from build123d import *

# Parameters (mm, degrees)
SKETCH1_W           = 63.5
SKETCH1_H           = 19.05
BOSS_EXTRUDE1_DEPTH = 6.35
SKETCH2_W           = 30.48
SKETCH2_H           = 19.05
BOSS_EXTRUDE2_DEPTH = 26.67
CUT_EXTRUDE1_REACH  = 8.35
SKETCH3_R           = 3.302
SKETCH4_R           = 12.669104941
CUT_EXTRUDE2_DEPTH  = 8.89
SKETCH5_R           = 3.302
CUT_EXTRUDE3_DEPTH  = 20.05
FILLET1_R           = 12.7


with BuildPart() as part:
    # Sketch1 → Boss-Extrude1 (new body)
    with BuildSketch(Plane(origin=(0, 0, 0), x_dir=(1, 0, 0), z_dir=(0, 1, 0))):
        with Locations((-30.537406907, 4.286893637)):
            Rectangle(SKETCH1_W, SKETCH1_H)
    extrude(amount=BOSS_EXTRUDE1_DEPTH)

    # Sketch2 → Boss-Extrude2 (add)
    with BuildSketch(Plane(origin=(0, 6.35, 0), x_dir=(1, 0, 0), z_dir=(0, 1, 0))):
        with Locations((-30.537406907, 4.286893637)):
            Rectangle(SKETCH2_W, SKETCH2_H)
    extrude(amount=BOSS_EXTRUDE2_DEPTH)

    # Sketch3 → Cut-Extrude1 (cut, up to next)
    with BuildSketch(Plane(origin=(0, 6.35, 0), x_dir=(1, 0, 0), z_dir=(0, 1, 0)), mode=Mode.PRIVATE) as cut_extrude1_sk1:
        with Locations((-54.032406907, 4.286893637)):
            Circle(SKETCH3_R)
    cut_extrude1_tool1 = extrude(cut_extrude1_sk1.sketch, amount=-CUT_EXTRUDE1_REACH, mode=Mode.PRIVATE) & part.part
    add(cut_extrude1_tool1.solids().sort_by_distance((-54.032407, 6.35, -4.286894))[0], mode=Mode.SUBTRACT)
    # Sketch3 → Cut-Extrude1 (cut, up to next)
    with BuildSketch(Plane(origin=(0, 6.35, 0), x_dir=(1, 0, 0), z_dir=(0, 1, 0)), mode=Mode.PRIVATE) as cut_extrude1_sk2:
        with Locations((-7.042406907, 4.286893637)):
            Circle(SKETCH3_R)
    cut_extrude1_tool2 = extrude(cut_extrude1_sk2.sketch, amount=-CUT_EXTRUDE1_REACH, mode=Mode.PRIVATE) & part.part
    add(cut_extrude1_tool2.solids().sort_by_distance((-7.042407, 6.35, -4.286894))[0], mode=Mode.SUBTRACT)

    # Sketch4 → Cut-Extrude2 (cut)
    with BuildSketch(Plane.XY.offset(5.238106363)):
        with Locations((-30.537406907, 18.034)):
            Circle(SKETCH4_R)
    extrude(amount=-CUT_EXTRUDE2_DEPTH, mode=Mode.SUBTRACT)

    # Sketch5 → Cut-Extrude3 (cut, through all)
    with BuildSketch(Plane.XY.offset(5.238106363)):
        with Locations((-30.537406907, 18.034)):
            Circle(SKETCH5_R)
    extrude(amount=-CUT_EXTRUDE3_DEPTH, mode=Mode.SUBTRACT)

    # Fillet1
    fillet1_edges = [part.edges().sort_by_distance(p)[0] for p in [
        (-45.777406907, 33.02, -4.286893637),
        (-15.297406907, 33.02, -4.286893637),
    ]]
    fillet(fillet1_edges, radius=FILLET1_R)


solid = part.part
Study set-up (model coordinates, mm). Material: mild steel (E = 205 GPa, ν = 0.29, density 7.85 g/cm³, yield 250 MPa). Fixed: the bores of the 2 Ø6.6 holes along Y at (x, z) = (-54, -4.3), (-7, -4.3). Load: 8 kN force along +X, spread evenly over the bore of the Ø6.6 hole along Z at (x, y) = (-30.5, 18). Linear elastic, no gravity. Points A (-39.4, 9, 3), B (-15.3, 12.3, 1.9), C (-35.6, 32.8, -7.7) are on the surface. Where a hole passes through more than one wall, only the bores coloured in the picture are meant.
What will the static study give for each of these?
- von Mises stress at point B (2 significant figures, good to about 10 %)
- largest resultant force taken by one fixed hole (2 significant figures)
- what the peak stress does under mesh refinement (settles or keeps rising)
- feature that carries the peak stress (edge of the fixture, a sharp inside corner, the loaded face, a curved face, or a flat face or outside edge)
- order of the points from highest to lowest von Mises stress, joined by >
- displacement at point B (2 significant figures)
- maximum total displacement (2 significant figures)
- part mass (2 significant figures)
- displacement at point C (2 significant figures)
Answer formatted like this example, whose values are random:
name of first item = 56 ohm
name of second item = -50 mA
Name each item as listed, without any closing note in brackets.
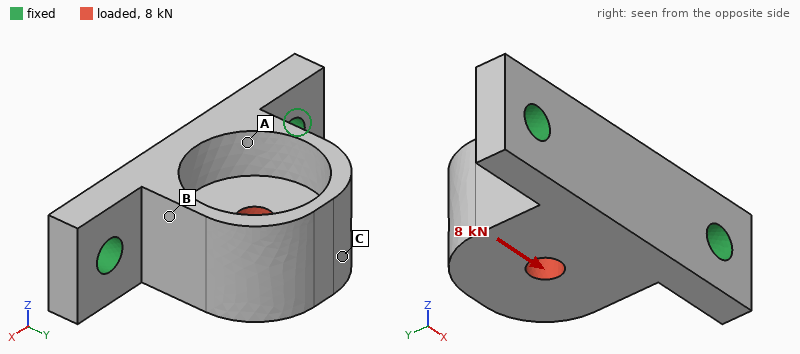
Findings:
von Mises stress at point B = 48 MPa
largest resultant force taken by one fixed hole = 5.2 kN
what the peak stress does under mesh refinement = keeps rising
feature that carries the peak stress = edge of the fixture
order of the points from highest to lowest von Mises stress, joined by > = B > A > C
displacement at point B = 7.5 µm
maximum total displacement = 22 µm
part mass = 130 g
displacement at point C = 20 µm
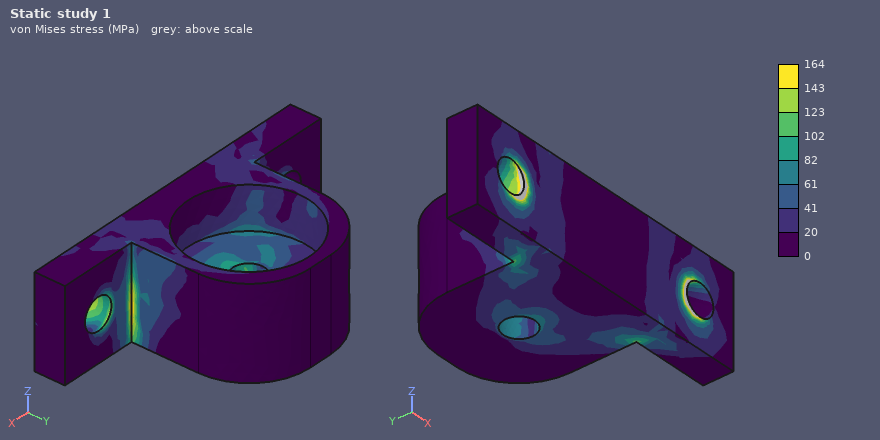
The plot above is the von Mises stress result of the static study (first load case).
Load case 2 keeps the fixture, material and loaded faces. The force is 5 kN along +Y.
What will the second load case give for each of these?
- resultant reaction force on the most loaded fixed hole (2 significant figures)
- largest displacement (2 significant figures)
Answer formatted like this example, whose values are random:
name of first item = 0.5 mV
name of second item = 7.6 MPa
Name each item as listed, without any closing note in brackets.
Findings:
resultant reaction force on the most loaded fixed hole = 2.7 kN
largest displacement = 27 µm
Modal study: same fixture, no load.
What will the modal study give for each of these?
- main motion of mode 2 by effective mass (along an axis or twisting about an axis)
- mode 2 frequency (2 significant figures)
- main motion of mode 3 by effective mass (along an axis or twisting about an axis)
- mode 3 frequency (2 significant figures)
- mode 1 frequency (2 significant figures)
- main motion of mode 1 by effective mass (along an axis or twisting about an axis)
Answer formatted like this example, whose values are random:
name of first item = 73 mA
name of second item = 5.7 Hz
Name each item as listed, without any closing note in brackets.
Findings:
main motion of mode 2 by effective mass = along X
mode 2 frequency = 12 kHz
main motion of mode 3 by effective mass = along Y
mode 3 frequency = 13 kHz
mode 1 frequency = 5000 Hz
main motion of mode 1 by effective mass = along Z
